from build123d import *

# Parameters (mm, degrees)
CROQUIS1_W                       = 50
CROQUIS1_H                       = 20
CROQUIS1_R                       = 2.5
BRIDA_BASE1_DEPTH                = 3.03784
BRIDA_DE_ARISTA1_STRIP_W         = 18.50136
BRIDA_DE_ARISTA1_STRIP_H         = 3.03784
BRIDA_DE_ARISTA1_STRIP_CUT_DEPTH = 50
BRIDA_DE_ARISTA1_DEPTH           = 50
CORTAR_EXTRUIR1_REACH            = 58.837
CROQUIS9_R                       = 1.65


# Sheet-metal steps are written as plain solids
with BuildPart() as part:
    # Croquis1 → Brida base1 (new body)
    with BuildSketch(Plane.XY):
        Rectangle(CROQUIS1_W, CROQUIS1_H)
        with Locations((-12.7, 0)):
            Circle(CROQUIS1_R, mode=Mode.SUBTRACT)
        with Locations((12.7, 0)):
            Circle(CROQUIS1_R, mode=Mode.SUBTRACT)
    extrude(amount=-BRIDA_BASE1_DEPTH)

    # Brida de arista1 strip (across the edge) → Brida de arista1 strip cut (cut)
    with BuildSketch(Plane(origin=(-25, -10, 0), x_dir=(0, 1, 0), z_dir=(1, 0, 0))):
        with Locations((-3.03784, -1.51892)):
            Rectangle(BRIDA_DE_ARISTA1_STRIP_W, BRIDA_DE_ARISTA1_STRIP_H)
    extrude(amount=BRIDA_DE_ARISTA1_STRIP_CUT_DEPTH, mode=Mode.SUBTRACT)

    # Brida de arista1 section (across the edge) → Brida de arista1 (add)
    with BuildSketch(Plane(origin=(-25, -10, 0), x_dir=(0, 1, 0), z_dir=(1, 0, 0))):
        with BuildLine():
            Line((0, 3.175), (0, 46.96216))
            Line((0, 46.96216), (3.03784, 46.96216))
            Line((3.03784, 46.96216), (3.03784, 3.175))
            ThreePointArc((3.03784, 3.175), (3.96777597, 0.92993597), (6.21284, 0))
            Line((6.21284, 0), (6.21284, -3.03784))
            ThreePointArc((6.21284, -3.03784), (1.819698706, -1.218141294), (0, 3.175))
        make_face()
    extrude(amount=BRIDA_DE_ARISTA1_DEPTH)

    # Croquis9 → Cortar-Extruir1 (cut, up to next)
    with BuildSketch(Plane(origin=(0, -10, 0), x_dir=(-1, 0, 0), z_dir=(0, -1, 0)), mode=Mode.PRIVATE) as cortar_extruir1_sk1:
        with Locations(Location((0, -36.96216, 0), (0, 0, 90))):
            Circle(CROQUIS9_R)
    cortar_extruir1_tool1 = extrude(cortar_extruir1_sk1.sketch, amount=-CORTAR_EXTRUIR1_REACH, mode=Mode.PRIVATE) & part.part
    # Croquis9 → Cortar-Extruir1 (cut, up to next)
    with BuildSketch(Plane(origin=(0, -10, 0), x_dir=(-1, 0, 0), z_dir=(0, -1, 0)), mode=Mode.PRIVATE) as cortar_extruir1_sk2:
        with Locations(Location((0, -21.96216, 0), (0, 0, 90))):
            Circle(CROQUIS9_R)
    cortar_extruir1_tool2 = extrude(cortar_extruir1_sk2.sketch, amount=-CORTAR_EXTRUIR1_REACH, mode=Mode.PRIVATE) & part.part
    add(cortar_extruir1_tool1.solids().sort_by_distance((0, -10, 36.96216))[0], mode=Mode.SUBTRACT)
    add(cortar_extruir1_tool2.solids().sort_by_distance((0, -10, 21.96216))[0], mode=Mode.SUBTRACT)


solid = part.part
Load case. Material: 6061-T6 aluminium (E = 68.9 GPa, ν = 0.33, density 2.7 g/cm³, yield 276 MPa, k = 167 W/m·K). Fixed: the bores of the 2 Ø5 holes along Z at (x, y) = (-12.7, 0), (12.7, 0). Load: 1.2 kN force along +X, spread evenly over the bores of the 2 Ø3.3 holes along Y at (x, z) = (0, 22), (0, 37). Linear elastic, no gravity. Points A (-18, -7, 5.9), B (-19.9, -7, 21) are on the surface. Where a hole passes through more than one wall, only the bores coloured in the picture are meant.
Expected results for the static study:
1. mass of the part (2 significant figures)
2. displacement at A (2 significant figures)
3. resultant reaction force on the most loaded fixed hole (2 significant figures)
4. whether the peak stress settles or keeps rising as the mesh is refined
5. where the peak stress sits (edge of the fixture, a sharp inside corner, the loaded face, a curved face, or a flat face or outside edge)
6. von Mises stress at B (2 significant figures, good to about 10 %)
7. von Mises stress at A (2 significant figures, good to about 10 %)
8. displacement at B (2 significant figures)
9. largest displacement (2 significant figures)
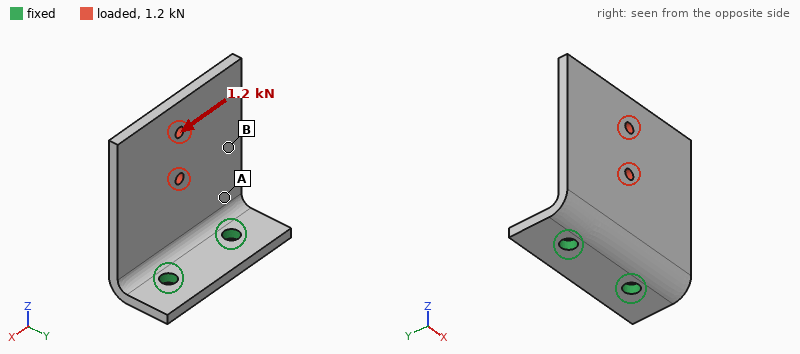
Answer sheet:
26 g
0.073 mm
1.5 kN
keeps rising
edge of the fixture
26 MPa
66 MPa
0.14 mm
0.24 mm
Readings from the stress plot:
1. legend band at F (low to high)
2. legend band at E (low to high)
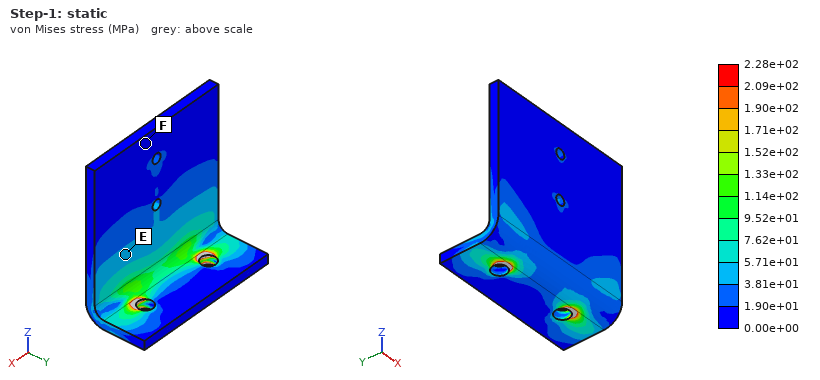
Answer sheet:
0.00e+00 to 1.90e+01 MPa
3.81e+01 to 5.71e+01 MPa
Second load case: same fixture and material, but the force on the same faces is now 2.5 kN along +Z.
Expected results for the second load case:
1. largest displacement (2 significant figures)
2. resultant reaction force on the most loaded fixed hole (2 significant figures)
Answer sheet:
0.51 mm
1.3 kN
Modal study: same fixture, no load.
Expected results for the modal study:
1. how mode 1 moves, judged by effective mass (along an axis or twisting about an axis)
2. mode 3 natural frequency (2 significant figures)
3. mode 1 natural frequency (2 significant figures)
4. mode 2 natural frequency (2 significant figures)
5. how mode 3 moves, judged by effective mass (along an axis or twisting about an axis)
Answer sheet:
along Y
4000 Hz
890 Hz
2200 Hz
along X
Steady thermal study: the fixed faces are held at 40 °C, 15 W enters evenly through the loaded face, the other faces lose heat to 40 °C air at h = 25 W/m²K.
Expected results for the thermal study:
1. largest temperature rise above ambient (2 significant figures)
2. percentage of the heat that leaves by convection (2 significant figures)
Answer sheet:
25 K
13 %
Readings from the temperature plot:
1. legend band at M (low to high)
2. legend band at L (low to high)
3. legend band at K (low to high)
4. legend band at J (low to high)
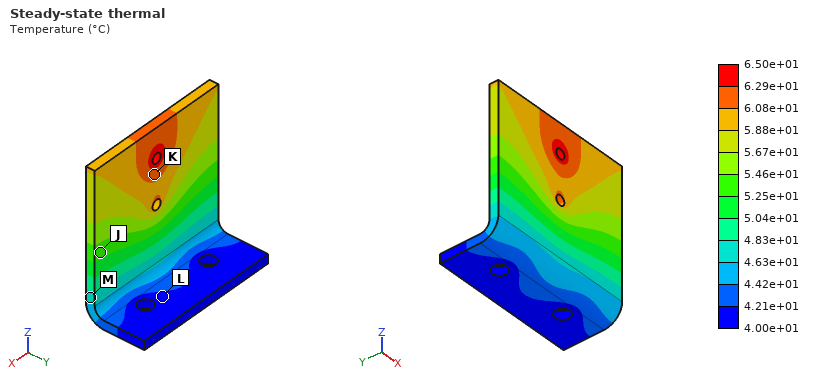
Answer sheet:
4.63e+01 to 4.83e+01 °C
4.00e+01 to 4.21e+01 °C
6.08e+01 to 6.29e+01 °C
5.25e+01 to 5.46e+01 °C
